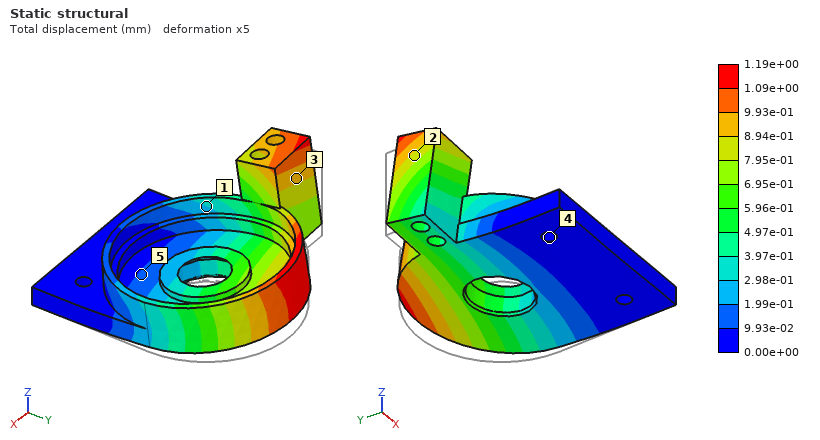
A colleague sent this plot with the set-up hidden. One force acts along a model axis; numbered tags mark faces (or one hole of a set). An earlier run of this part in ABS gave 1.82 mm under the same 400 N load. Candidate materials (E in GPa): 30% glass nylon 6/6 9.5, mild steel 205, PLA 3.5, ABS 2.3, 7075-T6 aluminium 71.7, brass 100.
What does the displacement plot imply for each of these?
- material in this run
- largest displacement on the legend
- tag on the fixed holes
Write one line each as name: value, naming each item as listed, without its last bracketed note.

material in this run: PLA
largest displacement on the legend: 1.19e+00 mm
tag on the fixed holes: 4
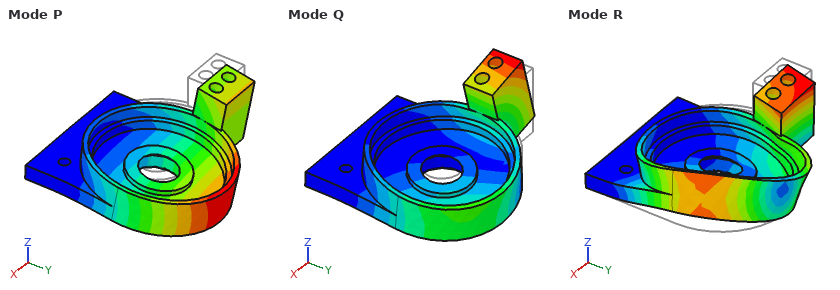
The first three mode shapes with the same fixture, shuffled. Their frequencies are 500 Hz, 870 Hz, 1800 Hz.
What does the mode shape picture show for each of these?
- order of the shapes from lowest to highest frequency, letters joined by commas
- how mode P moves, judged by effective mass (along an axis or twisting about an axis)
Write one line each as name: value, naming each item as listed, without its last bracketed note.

order of the shapes from lowest to highest frequency, letters joined by commas: P, Q, R
how mode P moves, judged by effective mass: along Z
